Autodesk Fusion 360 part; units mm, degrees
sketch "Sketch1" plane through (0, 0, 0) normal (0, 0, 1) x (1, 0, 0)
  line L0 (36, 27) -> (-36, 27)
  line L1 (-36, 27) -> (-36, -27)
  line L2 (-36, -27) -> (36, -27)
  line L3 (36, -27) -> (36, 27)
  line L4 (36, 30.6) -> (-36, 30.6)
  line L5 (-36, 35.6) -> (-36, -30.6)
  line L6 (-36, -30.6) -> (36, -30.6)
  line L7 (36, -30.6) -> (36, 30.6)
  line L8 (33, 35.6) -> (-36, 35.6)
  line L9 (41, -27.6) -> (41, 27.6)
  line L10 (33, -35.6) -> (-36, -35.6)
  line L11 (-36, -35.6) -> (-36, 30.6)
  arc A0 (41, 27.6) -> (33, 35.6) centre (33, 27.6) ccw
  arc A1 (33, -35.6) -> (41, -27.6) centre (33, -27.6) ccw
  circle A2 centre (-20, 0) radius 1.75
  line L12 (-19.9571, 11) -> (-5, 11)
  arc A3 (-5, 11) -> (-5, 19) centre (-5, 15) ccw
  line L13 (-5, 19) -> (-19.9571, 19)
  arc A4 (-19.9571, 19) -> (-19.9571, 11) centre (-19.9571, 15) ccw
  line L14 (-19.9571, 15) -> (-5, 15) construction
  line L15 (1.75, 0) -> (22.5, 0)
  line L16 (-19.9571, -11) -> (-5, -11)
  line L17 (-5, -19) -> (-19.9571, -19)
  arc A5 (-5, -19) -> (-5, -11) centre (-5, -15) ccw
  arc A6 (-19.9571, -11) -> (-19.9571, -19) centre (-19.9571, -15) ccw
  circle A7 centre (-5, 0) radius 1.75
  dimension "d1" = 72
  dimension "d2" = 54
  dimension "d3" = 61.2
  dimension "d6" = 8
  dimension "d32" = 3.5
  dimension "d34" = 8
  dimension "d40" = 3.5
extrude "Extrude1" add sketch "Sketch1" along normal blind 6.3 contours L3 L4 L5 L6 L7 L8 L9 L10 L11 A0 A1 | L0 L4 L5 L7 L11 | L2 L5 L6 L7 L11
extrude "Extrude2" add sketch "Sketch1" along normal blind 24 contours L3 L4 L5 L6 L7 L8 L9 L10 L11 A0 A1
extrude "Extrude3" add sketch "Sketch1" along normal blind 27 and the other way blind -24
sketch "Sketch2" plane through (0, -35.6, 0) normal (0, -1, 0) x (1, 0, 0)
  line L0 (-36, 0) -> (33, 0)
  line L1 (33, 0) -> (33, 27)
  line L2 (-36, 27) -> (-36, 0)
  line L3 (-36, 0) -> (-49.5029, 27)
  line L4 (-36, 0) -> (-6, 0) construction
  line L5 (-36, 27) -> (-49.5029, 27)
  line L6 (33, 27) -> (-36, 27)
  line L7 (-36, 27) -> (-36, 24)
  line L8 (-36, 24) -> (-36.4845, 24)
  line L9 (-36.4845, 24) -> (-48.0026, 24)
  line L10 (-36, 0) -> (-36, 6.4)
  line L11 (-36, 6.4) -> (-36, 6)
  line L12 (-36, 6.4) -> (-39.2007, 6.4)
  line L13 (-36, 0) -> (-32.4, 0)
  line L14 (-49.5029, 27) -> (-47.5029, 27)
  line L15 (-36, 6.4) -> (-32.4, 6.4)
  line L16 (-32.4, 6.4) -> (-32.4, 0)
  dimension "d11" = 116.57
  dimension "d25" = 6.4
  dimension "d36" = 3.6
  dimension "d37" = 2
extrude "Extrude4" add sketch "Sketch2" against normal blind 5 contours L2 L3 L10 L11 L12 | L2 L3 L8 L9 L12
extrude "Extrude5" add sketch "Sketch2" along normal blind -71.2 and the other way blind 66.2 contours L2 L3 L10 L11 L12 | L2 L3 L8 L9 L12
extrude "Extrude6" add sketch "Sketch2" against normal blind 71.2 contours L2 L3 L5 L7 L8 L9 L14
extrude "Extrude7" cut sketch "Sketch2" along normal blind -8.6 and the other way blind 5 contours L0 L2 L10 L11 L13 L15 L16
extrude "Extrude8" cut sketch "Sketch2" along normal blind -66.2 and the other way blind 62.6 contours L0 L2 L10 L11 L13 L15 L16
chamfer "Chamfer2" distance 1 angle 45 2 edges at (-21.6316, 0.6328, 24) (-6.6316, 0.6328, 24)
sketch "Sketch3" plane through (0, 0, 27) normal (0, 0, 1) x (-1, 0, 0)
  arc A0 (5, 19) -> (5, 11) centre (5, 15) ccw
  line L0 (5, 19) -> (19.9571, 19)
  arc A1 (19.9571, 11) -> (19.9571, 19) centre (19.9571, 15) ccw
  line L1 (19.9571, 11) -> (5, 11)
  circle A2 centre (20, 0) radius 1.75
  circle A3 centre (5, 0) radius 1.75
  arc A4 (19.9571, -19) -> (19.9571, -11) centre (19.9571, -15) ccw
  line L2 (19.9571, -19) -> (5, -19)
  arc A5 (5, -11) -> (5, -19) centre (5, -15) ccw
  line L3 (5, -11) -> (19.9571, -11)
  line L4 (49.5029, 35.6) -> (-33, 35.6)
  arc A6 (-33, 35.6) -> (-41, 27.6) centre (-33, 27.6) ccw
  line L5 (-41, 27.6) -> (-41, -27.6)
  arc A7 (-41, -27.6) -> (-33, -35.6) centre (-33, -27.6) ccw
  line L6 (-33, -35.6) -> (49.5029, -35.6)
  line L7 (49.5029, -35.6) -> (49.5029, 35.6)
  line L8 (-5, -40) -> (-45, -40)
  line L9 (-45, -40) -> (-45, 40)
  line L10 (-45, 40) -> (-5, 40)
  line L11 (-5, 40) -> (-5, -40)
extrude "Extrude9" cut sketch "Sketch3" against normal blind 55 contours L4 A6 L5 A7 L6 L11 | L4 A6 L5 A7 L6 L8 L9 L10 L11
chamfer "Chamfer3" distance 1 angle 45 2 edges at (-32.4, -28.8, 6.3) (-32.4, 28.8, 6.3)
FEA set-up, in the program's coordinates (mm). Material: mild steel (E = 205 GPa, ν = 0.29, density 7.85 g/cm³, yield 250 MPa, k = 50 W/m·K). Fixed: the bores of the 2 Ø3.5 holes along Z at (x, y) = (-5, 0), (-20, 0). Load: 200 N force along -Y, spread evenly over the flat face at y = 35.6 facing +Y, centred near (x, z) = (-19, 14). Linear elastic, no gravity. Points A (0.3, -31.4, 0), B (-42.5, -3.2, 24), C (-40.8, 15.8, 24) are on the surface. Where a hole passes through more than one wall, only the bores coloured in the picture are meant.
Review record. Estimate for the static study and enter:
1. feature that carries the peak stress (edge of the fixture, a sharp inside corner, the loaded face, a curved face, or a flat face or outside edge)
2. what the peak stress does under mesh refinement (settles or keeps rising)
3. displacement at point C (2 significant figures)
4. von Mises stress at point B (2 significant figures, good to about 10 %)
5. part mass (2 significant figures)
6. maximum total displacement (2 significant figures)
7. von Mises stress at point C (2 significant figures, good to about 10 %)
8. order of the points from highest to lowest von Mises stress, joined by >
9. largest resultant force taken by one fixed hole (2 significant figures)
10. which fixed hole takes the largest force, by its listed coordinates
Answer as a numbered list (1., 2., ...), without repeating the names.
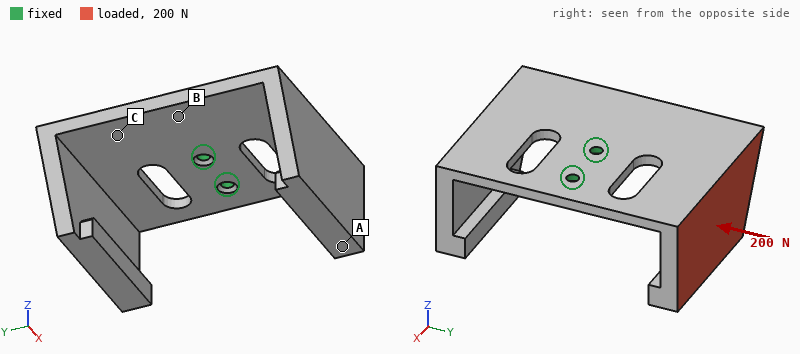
1. edge of the fixture
2. keeps rising
3. 0.031 mm
4. 17 MPa
5. 180 g
6. 0.16 mm
7. 37 MPa
8. C > B > A
9. 170 N
10. (-20, 0)
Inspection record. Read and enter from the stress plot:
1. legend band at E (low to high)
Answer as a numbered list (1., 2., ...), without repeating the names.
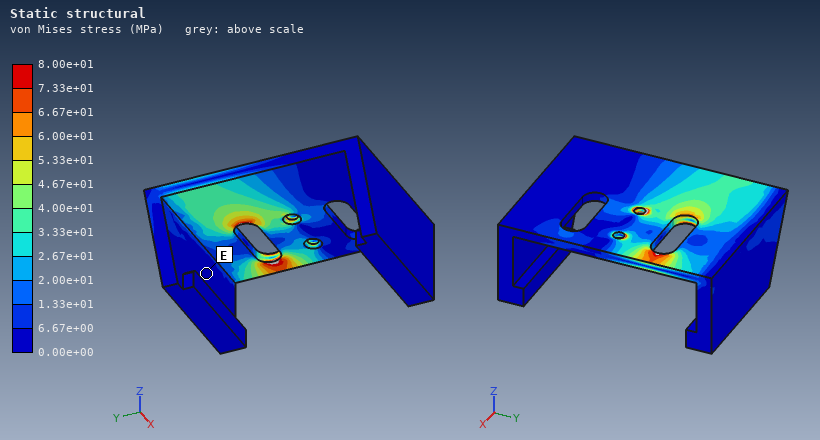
1. 0.00e+00 to 6.67e+00 MPa
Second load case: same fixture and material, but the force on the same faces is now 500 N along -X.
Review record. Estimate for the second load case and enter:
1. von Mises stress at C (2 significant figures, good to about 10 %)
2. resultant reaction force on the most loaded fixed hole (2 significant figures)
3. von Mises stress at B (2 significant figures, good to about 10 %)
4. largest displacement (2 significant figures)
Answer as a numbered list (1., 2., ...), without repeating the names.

1. 29 MPa
2. 1.1 kN
3. 29 MPa
4. 0.13 mm
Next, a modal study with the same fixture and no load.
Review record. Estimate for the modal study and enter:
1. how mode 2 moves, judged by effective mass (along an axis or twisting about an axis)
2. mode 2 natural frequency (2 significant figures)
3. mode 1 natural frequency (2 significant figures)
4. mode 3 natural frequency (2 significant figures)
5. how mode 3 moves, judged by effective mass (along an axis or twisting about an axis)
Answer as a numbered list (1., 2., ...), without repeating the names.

1. along Z
2. 650 Hz
3. 480 Hz
4. 1100 Hz
5. along X
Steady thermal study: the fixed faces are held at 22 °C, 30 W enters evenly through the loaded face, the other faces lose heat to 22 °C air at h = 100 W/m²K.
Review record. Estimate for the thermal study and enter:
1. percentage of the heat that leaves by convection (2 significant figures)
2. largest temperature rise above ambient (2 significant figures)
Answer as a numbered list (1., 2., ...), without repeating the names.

1. 84 %
2. 72 K
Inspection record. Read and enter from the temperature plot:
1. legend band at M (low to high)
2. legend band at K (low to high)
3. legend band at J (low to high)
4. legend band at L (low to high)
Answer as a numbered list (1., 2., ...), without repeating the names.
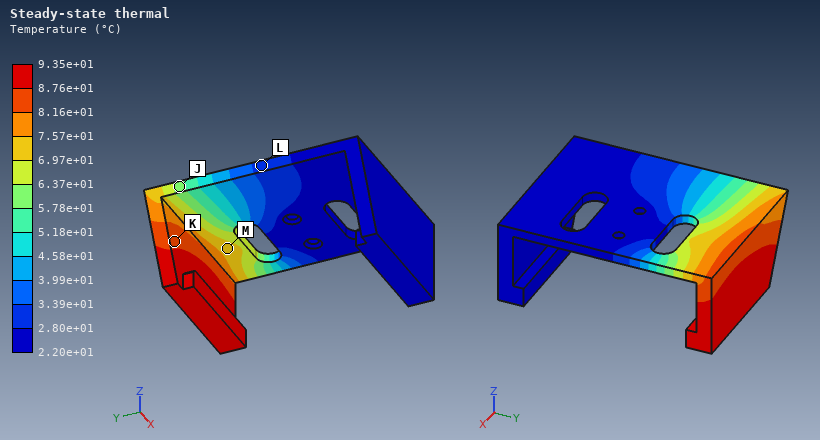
1. 6.97e+01 to 7.57e+01 °C
2. 8.16e+01 to 8.76e+01 °C
3. 5.78e+01 to 6.37e+01 °C
4. 2.80e+01 to 3.39e+01 °C
